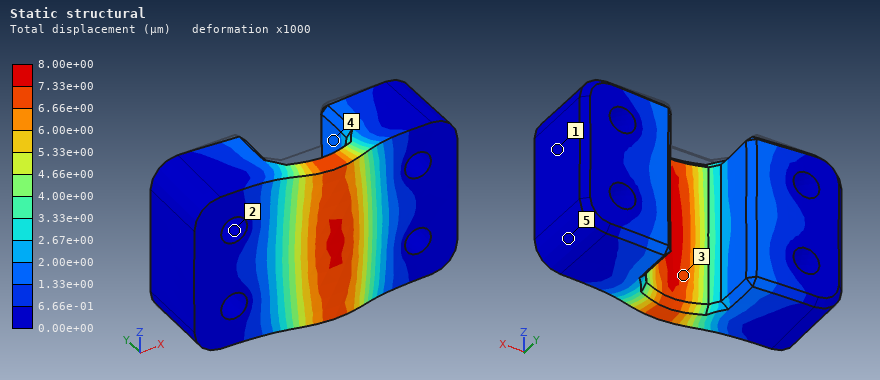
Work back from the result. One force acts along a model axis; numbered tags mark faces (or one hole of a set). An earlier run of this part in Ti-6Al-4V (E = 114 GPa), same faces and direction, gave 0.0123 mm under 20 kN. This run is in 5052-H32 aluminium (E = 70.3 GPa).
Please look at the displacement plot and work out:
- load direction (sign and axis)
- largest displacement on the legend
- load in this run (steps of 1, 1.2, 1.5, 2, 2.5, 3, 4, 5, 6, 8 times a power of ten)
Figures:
-Y
8.00e+00 µm
8 kN
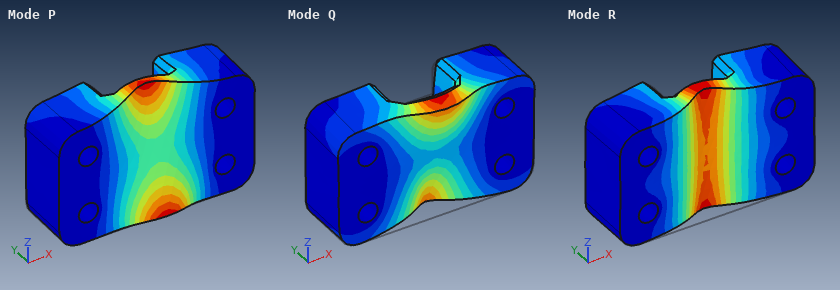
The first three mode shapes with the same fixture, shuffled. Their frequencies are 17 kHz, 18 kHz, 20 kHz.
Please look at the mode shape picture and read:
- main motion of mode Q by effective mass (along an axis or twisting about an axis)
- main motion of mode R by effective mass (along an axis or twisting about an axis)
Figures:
along Z
along Y
